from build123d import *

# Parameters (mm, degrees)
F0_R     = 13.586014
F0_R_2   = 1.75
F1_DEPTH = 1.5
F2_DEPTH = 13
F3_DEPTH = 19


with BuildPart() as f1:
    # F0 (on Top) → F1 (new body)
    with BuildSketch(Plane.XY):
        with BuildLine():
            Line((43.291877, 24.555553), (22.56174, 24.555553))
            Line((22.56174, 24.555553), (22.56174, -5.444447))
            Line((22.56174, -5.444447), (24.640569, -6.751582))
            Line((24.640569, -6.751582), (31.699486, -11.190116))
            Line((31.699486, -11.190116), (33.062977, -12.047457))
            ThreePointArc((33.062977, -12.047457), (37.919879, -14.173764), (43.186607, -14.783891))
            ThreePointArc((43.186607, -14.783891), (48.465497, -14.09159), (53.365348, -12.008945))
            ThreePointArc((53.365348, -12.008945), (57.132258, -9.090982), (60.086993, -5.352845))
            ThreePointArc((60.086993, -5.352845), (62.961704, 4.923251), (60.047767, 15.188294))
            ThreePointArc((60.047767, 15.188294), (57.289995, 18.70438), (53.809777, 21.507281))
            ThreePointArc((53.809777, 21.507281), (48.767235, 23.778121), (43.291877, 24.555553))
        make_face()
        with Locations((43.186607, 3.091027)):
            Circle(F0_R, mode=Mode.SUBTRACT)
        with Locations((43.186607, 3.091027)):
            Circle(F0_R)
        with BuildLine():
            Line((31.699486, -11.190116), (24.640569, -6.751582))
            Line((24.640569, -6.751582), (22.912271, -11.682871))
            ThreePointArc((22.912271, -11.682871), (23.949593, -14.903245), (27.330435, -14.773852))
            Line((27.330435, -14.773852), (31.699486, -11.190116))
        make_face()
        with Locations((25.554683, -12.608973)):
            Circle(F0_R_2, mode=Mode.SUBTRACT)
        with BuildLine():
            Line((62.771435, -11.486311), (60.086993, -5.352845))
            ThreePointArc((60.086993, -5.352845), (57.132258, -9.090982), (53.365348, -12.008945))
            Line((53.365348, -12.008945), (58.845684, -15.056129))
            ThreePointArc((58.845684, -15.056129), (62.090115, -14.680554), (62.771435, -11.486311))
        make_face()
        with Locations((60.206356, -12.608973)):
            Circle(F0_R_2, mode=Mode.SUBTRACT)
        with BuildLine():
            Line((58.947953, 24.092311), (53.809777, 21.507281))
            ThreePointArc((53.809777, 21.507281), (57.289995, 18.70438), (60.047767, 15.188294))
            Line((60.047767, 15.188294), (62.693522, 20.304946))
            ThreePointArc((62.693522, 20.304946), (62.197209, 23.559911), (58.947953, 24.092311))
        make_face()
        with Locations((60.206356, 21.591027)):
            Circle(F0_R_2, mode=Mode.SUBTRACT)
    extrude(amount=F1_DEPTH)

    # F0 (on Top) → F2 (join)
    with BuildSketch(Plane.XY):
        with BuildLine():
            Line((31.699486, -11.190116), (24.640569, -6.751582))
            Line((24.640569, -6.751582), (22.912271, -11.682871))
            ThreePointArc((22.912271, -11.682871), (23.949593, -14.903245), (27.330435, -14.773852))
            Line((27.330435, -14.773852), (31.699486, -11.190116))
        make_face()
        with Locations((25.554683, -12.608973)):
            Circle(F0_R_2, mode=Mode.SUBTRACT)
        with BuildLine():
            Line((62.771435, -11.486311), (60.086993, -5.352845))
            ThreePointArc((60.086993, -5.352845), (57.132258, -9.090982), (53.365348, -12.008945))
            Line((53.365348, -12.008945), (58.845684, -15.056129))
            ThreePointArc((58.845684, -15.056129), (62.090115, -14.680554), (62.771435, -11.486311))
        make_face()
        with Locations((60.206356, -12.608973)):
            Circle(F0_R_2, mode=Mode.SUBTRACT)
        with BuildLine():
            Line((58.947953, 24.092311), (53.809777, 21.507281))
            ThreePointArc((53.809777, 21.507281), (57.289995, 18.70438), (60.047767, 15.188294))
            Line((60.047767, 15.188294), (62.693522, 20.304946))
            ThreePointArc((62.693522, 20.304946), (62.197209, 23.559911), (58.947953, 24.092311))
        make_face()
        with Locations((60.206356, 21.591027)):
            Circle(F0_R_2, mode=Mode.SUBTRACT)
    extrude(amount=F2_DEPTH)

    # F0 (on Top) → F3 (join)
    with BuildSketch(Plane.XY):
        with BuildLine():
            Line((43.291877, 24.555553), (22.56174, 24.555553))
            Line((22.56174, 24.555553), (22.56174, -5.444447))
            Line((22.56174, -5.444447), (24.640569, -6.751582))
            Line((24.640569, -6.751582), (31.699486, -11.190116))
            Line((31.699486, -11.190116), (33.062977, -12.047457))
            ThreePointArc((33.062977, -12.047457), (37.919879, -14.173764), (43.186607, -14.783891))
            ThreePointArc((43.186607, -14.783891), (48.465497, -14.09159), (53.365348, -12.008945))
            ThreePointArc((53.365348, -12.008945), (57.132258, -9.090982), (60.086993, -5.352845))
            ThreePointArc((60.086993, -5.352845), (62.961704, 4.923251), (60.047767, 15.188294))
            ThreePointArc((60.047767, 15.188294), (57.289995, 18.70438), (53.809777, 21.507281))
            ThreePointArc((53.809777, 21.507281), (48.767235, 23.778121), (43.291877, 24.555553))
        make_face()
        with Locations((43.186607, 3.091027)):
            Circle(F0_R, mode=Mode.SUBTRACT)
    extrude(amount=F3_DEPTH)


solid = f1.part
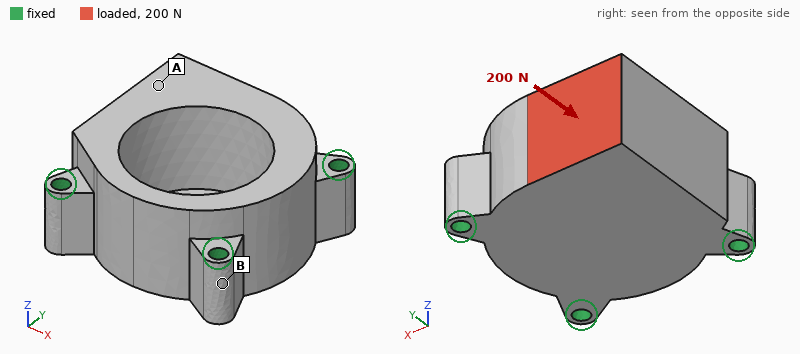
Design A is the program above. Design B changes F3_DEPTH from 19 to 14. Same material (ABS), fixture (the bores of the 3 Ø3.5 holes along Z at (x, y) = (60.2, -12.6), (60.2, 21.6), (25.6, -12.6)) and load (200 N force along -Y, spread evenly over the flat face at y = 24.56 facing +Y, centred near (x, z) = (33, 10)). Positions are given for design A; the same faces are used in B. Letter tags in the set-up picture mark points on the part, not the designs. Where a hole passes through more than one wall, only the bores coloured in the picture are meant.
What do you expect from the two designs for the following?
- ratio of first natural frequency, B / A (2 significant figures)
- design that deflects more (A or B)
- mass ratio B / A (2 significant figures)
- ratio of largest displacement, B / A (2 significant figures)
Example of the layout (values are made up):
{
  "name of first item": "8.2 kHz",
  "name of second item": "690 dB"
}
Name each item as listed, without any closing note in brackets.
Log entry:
{
  "ratio of first natural frequency, B / A": "1.1",
  "design that deflects more": "A",
  "mass ratio B / A": "0.77",
  "ratio of largest displacement, B / A": "0.92"
}
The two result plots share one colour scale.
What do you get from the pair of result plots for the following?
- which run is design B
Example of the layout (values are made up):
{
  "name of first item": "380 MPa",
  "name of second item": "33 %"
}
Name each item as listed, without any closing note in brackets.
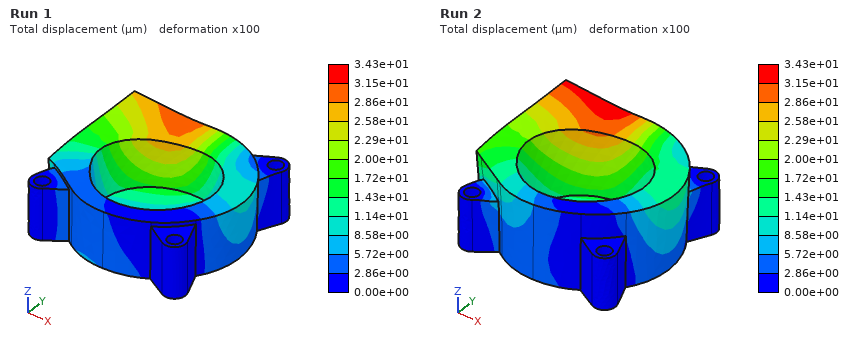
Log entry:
{
  "which run is design B": "Run 1"
}
